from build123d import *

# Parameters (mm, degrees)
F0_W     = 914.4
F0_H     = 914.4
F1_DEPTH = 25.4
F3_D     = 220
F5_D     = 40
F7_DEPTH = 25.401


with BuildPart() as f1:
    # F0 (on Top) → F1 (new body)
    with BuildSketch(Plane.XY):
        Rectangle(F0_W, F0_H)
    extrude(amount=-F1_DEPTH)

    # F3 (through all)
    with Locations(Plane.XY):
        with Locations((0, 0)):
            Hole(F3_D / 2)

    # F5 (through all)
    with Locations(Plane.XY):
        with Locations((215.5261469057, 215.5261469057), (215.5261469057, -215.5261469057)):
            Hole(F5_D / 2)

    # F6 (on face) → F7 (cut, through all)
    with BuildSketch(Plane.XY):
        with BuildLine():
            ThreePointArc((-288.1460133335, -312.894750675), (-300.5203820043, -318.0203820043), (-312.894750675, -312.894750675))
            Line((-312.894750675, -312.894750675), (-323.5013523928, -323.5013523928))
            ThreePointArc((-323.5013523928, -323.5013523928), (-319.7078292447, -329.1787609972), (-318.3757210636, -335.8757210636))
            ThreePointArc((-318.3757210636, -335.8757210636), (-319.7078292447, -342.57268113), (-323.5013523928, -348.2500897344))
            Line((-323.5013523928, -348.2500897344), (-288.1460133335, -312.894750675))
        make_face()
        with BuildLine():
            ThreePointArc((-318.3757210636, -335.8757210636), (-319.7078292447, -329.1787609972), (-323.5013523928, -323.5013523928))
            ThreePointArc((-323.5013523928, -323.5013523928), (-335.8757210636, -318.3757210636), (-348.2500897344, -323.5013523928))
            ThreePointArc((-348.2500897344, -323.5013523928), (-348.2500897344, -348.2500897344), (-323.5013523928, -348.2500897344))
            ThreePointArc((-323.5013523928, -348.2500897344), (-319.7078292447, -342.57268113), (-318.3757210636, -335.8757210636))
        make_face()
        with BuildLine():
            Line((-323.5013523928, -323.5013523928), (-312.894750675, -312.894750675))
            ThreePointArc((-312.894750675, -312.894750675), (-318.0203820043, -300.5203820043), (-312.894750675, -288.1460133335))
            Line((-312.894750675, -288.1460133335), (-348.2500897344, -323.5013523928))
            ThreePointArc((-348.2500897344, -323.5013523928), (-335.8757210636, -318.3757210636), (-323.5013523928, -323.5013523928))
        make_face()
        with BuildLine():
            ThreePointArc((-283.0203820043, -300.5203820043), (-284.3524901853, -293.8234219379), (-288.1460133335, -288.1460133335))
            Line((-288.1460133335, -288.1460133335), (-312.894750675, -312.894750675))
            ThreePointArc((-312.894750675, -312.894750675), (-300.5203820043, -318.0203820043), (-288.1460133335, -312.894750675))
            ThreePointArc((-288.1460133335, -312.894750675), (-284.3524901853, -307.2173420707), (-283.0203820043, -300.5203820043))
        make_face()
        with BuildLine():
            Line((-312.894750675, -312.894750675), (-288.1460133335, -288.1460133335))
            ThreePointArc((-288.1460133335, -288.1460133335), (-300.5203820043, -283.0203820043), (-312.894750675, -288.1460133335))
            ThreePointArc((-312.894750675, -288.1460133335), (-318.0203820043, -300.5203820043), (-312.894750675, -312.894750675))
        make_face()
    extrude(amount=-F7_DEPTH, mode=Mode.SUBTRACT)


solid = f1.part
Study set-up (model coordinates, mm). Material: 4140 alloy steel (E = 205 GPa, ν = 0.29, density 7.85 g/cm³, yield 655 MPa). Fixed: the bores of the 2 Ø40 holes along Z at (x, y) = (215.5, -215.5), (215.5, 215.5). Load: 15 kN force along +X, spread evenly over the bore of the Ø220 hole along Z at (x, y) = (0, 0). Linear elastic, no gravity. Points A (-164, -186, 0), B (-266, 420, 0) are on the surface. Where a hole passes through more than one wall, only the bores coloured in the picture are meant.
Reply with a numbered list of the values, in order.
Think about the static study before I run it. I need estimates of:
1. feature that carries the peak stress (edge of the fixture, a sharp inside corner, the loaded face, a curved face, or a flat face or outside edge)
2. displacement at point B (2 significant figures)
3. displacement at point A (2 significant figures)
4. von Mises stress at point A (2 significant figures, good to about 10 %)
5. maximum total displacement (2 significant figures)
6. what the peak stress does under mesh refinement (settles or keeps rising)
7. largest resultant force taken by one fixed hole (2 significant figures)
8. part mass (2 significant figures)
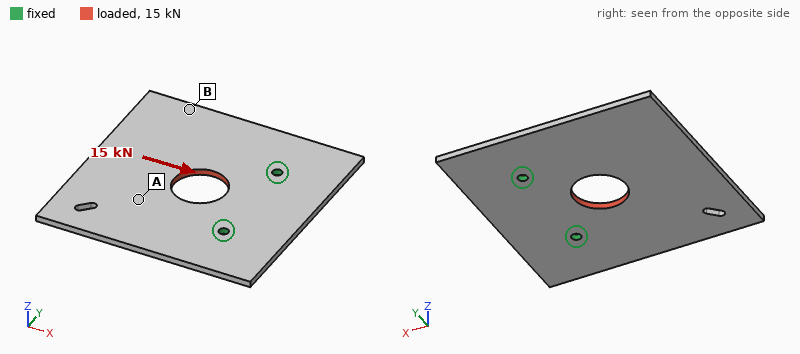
1. edge of the fixture
2. 1.0 µm
3. 1.6 µm
4. 0.47 MPa
5. 2.5 µm
6. keeps rising
7. 7.6 kN
8. 160 kg
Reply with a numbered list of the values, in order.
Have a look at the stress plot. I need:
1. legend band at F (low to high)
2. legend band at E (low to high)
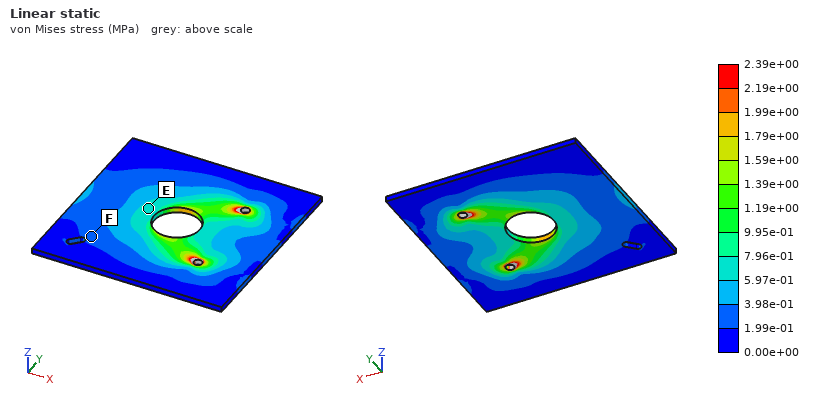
1. 1.99e-01 to 3.98e-01 MPa
2. 5.97e-01 to 7.96e-01 MPa
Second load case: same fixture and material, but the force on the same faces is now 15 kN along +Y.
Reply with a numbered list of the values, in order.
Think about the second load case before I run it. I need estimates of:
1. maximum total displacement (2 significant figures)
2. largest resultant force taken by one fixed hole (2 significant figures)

1. 8.9 µm
2. 10 kN
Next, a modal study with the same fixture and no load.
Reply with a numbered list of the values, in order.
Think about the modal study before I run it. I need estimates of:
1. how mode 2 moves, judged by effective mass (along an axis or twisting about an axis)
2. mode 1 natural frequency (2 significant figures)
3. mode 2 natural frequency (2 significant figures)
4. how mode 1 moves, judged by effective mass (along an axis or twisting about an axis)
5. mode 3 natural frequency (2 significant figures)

1. twisting about X
2. 41 Hz
3. 80 Hz
4. along Z
5. 190 Hz
